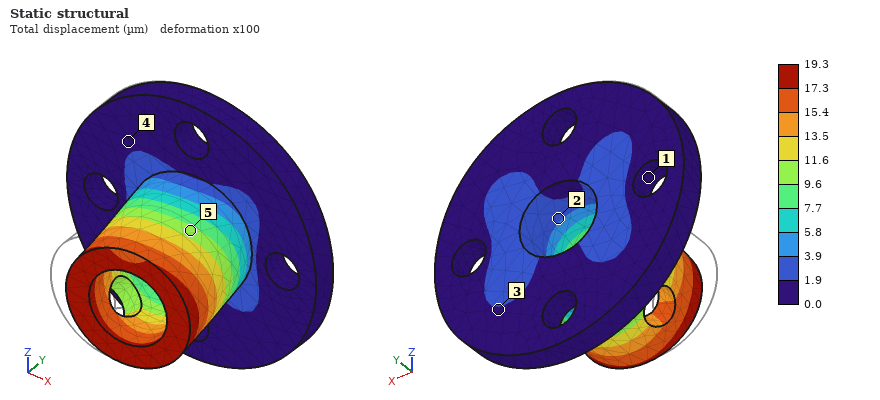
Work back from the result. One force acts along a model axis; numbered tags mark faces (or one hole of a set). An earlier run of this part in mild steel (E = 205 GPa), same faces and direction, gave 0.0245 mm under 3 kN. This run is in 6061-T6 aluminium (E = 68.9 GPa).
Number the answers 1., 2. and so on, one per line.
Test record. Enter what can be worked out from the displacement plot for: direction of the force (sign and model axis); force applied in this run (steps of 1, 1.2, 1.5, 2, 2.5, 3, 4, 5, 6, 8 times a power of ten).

1. +X
2. 800 N
